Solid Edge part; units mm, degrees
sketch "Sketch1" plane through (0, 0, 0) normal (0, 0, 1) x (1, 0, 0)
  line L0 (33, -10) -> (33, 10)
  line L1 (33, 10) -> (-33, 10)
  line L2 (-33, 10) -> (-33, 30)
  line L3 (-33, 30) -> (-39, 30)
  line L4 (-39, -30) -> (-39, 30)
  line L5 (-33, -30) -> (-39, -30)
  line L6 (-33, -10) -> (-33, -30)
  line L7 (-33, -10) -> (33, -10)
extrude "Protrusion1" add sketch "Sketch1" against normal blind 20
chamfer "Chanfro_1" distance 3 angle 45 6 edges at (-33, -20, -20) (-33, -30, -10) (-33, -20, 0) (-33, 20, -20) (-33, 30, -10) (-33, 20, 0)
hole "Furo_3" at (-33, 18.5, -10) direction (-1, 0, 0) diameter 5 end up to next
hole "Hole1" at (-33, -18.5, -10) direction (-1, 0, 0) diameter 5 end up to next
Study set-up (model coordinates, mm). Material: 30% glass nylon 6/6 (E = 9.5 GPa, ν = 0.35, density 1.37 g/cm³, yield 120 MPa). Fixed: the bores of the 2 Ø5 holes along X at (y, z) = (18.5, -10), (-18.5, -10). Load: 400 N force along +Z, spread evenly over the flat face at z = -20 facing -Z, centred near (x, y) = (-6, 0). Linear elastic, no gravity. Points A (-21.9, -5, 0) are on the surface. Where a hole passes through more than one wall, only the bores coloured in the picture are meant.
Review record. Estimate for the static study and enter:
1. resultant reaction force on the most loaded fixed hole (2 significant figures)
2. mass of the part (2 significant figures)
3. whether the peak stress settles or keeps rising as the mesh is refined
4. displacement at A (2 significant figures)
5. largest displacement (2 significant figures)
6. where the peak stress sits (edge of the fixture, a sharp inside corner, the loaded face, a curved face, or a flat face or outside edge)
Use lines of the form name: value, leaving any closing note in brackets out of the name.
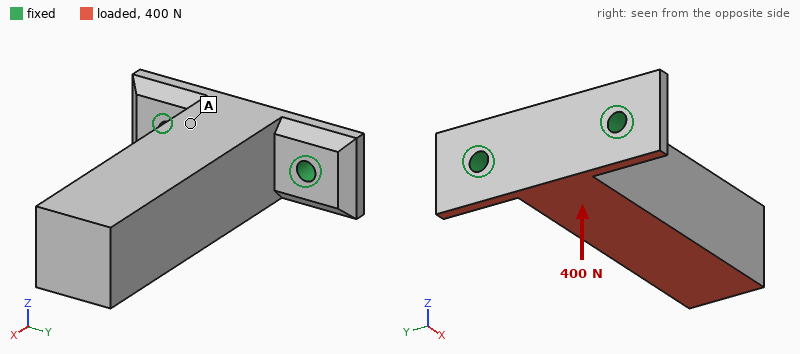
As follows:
resultant reaction force on the most loaded fixed hole: 200 N
mass of the part: 45 g
whether the peak stress settles or keeps rising as the mesh is refined: keeps rising
displacement at A: 0.23 mm
largest displacement: 0.97 mm
where the peak stress sits: edge of the fixture
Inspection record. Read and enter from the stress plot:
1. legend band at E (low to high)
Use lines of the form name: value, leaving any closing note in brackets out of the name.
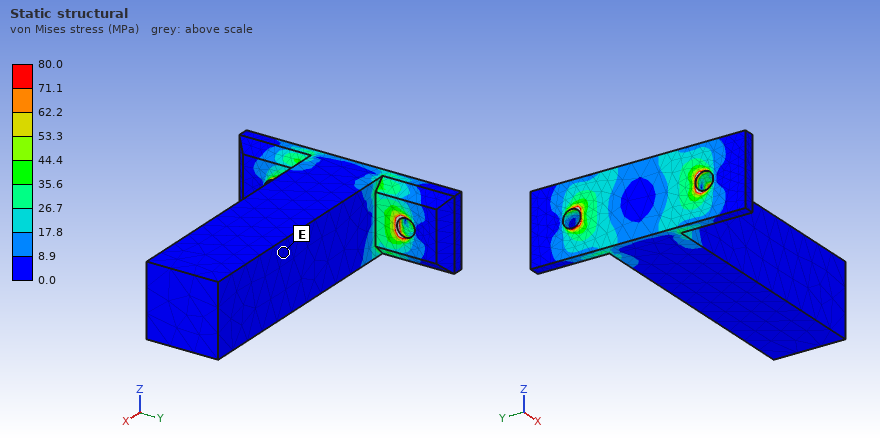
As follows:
legend band at E: 0.0 to 8.9 MPa
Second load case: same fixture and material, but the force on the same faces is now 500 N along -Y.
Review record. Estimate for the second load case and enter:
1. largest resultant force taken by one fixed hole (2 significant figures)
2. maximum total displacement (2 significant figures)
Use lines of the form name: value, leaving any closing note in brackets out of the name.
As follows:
largest resultant force taken by one fixed hole: 610 N
maximum total displacement: 0.33 mm
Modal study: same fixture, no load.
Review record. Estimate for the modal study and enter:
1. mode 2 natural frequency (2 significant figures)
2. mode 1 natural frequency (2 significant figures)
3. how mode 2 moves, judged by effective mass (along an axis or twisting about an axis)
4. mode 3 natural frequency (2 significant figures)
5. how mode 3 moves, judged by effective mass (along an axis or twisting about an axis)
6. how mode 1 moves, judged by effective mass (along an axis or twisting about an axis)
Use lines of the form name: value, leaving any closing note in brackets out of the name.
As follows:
mode 2 natural frequency: 1200 Hz
mode 1 natural frequency: 600 Hz
how mode 2 moves, judged by effective mass: along Y
mode 3 natural frequency: 4100 Hz
how mode 3 moves, judged by effective mass: along X
how mode 1 moves, judged by effective mass: along Z
